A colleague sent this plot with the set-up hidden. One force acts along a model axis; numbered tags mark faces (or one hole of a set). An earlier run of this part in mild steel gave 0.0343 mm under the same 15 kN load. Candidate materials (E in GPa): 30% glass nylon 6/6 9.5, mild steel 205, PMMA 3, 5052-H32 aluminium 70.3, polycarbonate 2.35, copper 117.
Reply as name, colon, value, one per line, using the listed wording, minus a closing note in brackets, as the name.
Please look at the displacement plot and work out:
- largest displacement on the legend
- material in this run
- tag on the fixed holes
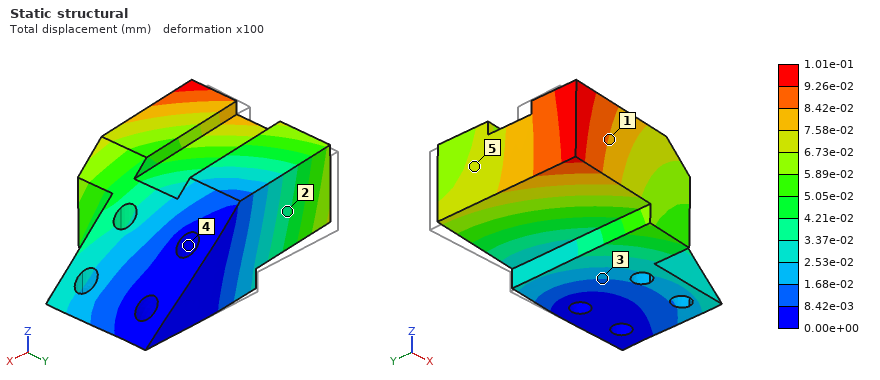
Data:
largest displacement on the legend: 1.01e-01 mm
material in this run: 5052-H32 aluminium
tag on the fixed holes: 4
